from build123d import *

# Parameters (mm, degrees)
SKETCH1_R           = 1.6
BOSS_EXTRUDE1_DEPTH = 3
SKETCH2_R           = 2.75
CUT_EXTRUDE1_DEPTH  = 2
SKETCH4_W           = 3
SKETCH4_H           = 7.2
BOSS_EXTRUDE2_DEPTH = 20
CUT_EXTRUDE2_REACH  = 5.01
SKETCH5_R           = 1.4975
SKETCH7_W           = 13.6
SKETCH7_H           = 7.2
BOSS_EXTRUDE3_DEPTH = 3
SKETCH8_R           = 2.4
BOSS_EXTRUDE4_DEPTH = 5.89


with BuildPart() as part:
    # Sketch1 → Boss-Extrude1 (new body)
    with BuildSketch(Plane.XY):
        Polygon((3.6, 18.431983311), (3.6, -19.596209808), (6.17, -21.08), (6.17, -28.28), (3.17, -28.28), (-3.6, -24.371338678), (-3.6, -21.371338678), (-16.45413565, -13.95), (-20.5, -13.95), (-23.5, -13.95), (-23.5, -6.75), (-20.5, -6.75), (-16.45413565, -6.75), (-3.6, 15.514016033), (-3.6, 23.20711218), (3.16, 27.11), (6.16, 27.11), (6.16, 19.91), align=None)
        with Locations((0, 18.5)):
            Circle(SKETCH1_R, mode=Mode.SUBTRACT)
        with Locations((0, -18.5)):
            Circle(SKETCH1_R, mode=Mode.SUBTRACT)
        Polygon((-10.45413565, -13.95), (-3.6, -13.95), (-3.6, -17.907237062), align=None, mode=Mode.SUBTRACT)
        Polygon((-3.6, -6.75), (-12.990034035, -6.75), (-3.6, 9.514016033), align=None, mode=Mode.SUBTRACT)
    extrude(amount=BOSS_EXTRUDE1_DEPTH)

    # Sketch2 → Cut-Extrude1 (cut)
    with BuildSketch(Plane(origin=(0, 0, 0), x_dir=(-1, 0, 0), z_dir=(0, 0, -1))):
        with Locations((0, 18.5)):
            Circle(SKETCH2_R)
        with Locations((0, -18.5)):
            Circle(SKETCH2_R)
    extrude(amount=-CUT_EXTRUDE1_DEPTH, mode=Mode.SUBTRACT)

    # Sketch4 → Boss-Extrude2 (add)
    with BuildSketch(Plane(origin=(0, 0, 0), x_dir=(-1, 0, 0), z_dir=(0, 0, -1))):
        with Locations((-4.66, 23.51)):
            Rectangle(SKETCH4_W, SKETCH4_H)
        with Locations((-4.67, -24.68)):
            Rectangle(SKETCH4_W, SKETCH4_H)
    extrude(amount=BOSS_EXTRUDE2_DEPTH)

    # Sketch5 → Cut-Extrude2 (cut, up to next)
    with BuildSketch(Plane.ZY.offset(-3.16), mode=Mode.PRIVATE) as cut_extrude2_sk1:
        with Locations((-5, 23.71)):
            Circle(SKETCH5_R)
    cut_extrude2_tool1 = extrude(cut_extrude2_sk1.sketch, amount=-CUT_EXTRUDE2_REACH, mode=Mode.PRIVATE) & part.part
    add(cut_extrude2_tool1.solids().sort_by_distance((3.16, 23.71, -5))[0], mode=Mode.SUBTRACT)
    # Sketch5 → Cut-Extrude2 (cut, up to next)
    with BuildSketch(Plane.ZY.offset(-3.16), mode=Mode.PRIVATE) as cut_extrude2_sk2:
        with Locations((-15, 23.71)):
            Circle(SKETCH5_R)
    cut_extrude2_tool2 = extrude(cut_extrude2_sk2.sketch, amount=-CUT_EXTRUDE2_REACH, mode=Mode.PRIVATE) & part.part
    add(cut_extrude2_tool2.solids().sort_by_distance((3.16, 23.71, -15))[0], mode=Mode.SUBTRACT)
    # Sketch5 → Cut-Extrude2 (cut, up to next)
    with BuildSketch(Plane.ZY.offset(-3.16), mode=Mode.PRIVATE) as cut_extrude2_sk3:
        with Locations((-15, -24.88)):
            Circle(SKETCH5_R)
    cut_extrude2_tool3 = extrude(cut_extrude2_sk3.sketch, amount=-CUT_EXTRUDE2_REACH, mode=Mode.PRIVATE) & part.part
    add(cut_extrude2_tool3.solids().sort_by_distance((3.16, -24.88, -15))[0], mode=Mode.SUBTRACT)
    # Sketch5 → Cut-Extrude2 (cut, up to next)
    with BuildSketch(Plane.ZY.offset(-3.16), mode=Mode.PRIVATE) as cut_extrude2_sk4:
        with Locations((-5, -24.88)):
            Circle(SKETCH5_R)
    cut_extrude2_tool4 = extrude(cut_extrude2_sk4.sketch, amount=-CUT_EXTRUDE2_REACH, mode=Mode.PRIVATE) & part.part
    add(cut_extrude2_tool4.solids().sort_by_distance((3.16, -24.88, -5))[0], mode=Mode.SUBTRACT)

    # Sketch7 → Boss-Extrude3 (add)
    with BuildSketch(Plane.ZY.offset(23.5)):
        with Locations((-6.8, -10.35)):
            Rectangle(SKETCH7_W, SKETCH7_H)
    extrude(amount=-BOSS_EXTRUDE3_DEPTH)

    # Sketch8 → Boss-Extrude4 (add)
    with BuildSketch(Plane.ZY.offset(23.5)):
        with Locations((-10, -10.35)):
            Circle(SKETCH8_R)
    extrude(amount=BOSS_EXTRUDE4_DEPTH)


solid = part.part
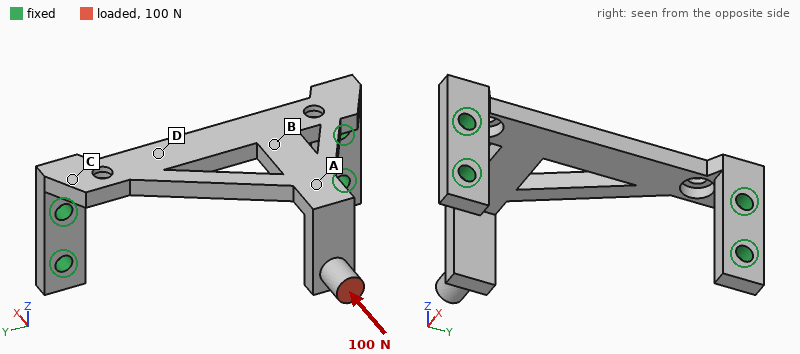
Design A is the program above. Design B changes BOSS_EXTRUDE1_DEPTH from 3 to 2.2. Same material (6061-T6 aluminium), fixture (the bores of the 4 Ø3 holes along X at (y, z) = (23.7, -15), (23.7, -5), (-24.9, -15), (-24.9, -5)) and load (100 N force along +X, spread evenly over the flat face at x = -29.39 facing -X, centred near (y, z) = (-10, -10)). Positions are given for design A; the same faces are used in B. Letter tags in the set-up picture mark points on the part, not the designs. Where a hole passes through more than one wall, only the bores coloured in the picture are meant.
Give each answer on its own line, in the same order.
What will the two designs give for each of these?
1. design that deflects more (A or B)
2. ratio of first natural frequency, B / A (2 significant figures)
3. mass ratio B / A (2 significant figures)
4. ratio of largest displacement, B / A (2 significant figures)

B
0.73
0.83
2.1
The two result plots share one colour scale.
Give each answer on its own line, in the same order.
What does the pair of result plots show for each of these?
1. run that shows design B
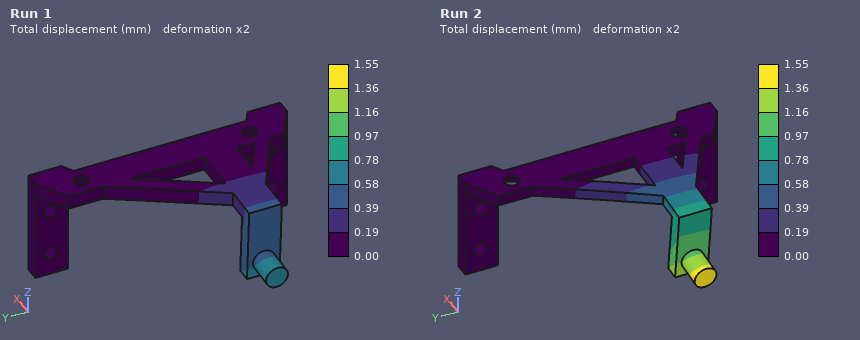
Run 2
